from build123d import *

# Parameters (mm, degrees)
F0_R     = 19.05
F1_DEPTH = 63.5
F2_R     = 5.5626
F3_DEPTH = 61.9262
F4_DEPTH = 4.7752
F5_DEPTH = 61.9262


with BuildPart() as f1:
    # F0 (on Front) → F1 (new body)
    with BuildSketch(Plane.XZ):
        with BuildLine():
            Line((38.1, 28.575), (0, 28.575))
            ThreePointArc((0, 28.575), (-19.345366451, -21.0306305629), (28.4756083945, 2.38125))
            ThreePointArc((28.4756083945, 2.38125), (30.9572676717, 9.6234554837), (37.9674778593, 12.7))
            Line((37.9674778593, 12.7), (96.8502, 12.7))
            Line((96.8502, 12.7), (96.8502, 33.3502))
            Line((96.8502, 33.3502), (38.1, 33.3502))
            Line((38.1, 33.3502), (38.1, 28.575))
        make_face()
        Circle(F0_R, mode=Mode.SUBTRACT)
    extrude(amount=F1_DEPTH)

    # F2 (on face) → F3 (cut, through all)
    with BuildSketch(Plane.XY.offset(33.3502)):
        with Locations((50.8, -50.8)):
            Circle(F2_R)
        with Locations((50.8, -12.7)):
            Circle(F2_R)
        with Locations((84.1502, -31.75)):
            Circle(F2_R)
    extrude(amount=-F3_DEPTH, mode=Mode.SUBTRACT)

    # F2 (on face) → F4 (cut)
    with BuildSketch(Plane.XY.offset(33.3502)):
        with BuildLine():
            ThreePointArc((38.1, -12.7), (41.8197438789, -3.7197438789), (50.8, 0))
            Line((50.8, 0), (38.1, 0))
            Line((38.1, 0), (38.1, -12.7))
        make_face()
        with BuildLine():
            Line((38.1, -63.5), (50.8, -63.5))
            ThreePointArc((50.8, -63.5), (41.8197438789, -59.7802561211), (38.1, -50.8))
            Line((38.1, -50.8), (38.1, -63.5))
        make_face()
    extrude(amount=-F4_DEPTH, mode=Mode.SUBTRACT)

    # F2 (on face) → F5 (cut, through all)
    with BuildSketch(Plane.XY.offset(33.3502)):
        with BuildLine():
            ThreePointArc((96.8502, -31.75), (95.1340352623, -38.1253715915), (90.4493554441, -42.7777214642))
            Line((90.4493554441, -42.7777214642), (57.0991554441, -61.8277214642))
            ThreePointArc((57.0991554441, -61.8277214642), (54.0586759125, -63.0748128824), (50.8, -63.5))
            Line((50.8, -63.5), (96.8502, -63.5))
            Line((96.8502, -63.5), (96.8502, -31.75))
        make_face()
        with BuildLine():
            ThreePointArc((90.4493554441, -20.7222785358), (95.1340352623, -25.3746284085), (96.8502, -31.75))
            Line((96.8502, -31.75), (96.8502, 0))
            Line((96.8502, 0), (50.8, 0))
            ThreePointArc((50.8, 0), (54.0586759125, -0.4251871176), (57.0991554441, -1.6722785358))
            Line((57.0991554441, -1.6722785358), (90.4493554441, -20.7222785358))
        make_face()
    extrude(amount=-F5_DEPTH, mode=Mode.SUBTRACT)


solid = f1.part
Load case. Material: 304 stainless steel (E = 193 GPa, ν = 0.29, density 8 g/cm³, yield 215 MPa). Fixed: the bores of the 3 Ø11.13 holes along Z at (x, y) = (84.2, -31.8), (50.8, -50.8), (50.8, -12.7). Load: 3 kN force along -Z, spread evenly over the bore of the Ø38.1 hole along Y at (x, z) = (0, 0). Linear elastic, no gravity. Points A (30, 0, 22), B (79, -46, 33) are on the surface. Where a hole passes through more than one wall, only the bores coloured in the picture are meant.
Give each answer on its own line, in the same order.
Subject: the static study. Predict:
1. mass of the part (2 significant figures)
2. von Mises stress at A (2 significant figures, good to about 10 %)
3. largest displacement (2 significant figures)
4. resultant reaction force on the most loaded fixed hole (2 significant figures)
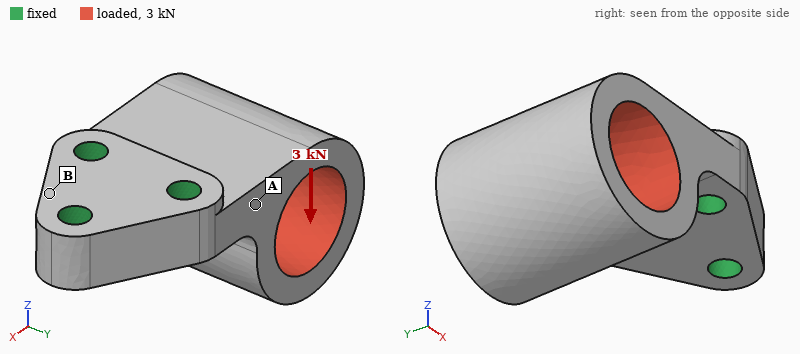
1.3 kg
14 MPa
48 µm
1.8 kN
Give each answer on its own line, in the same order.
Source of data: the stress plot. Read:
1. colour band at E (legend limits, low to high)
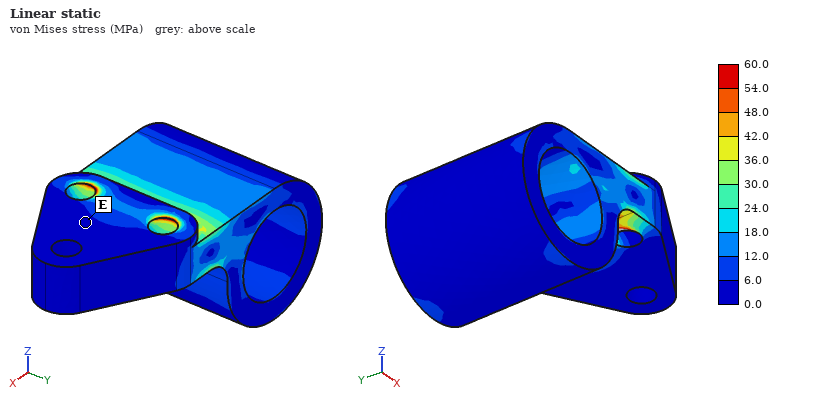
0.0 to 6.0 MPa
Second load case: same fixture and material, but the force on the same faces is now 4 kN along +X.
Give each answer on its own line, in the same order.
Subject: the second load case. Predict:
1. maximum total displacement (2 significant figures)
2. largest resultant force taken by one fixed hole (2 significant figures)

39 µm
1.9 kN
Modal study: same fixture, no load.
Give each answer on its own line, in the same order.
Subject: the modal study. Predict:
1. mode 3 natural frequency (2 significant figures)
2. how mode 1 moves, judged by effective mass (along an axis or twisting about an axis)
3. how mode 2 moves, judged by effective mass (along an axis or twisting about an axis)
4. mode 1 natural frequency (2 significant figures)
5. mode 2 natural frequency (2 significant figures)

5800 Hz
along Z
along Y
1500 Hz
3600 Hz
